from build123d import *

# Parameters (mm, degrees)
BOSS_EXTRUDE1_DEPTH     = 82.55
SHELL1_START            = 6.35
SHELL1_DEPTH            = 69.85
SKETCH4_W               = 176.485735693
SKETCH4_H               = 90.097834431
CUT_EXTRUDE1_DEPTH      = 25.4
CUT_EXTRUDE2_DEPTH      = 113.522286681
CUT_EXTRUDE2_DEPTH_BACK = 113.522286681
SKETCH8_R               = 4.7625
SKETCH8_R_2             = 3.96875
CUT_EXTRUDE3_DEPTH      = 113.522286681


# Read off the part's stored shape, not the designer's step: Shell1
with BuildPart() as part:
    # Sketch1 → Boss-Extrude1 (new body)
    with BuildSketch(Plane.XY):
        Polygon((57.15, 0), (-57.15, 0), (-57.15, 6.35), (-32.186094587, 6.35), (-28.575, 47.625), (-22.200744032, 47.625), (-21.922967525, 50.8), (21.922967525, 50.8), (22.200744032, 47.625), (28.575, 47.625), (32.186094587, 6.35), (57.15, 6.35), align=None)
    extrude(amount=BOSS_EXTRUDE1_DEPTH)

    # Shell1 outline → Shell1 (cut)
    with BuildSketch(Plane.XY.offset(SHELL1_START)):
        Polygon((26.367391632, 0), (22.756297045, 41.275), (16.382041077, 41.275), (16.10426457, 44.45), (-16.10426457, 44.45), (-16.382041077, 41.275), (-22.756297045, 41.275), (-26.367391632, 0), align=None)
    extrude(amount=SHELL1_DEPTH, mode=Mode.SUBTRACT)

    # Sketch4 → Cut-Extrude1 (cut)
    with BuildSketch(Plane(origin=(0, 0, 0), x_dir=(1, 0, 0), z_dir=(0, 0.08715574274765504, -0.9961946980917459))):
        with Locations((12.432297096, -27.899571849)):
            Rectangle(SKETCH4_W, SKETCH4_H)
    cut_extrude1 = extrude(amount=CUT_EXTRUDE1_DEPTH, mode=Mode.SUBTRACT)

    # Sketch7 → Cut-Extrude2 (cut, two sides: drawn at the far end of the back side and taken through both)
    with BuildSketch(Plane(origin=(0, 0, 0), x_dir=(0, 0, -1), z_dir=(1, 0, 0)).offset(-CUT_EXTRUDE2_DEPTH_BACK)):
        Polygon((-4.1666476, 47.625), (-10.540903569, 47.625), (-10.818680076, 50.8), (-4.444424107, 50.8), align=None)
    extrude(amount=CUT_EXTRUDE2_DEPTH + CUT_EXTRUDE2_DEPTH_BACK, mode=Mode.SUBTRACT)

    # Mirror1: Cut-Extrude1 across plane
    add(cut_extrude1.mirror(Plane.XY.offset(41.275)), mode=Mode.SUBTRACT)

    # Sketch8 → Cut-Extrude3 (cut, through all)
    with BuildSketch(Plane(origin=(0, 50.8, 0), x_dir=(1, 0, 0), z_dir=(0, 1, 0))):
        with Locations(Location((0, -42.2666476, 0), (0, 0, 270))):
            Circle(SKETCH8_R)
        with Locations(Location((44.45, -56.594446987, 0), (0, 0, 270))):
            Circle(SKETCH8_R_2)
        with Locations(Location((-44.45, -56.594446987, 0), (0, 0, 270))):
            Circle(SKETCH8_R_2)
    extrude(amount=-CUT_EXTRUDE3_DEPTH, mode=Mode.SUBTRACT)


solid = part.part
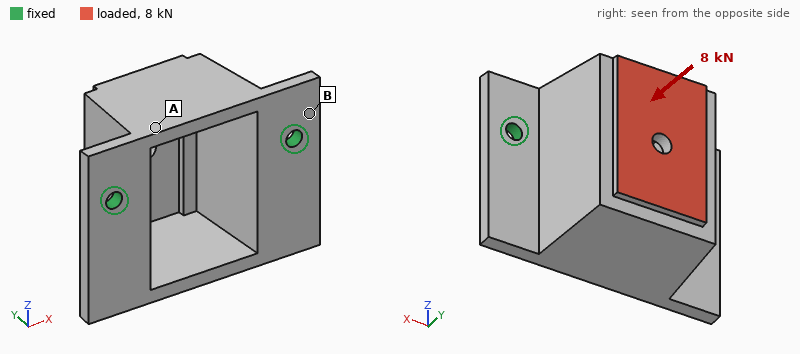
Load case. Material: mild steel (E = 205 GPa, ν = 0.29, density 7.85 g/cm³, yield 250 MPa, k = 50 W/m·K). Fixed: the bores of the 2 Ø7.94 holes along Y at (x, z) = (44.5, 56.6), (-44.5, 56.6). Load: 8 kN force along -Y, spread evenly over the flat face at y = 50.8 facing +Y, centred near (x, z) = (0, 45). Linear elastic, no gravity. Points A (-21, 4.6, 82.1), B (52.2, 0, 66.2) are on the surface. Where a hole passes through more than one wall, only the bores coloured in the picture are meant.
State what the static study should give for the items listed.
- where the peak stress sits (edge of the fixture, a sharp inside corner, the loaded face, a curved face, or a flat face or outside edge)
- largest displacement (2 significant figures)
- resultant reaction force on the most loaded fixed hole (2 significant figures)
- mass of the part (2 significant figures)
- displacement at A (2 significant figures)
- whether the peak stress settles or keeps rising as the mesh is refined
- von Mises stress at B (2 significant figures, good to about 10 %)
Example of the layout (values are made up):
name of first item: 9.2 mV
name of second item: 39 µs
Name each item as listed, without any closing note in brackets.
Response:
where the peak stress sits: edge of the fixture
largest displacement: 0.13 mm
resultant reaction force on the most loaded fixed hole: 4.3 kN
mass of the part: 900 g
displacement at A: 0.027 mm
whether the peak stress settles or keeps rising as the mesh is refined: keeps rising
von Mises stress at B: 38 MPa
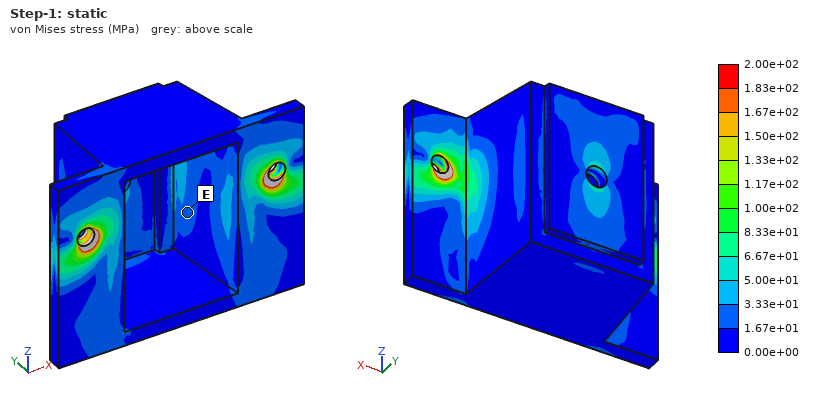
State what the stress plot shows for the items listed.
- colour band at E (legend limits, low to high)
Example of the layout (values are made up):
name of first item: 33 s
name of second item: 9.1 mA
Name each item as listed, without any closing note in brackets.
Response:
colour band at E: 1.67e+01 to 3.33e+01 MPa
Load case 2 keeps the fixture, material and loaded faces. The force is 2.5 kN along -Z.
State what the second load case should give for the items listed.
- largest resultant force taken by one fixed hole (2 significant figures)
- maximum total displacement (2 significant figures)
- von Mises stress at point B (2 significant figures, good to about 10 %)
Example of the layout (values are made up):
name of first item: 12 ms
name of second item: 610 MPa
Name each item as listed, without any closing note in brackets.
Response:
largest resultant force taken by one fixed hole: 1.3 kN
maximum total displacement: 0.15 mm
von Mises stress at point B: 77 MPa
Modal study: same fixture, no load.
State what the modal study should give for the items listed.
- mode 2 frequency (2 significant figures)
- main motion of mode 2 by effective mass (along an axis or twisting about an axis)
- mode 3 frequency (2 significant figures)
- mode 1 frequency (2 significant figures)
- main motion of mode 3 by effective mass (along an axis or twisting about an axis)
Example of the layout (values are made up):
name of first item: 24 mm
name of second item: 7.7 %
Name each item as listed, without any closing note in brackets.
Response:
mode 2 frequency: 3000 Hz
main motion of mode 2 by effective mass: along X
mode 3 frequency: 3600 Hz
mode 1 frequency: 1000 Hz
main motion of mode 3 by effective mass: along X
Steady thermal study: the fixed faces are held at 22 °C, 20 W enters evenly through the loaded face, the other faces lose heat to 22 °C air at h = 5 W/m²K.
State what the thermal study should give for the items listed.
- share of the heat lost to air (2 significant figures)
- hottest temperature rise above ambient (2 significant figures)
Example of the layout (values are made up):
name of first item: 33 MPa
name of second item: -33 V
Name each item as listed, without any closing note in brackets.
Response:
share of the heat lost to air: 16 %
hottest temperature rise above ambient: 28 K
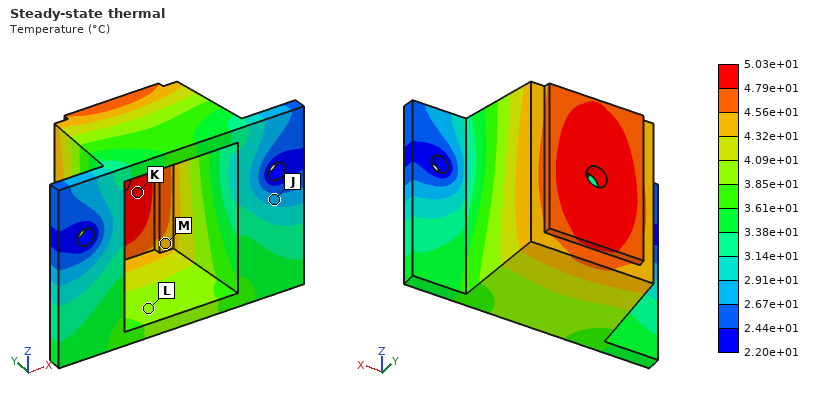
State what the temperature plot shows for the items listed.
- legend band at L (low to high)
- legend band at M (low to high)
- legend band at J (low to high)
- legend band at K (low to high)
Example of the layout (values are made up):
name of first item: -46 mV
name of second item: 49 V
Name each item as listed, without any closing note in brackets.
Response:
legend band at L: 3.85e+01 to 4.09e+01 °C
legend band at M: 4.32e+01 to 4.56e+01 °C
legend band at J: 2.67e+01 to 2.91e+01 °C
legend band at K: 4.79e+01 to 5.03e+01 °C
